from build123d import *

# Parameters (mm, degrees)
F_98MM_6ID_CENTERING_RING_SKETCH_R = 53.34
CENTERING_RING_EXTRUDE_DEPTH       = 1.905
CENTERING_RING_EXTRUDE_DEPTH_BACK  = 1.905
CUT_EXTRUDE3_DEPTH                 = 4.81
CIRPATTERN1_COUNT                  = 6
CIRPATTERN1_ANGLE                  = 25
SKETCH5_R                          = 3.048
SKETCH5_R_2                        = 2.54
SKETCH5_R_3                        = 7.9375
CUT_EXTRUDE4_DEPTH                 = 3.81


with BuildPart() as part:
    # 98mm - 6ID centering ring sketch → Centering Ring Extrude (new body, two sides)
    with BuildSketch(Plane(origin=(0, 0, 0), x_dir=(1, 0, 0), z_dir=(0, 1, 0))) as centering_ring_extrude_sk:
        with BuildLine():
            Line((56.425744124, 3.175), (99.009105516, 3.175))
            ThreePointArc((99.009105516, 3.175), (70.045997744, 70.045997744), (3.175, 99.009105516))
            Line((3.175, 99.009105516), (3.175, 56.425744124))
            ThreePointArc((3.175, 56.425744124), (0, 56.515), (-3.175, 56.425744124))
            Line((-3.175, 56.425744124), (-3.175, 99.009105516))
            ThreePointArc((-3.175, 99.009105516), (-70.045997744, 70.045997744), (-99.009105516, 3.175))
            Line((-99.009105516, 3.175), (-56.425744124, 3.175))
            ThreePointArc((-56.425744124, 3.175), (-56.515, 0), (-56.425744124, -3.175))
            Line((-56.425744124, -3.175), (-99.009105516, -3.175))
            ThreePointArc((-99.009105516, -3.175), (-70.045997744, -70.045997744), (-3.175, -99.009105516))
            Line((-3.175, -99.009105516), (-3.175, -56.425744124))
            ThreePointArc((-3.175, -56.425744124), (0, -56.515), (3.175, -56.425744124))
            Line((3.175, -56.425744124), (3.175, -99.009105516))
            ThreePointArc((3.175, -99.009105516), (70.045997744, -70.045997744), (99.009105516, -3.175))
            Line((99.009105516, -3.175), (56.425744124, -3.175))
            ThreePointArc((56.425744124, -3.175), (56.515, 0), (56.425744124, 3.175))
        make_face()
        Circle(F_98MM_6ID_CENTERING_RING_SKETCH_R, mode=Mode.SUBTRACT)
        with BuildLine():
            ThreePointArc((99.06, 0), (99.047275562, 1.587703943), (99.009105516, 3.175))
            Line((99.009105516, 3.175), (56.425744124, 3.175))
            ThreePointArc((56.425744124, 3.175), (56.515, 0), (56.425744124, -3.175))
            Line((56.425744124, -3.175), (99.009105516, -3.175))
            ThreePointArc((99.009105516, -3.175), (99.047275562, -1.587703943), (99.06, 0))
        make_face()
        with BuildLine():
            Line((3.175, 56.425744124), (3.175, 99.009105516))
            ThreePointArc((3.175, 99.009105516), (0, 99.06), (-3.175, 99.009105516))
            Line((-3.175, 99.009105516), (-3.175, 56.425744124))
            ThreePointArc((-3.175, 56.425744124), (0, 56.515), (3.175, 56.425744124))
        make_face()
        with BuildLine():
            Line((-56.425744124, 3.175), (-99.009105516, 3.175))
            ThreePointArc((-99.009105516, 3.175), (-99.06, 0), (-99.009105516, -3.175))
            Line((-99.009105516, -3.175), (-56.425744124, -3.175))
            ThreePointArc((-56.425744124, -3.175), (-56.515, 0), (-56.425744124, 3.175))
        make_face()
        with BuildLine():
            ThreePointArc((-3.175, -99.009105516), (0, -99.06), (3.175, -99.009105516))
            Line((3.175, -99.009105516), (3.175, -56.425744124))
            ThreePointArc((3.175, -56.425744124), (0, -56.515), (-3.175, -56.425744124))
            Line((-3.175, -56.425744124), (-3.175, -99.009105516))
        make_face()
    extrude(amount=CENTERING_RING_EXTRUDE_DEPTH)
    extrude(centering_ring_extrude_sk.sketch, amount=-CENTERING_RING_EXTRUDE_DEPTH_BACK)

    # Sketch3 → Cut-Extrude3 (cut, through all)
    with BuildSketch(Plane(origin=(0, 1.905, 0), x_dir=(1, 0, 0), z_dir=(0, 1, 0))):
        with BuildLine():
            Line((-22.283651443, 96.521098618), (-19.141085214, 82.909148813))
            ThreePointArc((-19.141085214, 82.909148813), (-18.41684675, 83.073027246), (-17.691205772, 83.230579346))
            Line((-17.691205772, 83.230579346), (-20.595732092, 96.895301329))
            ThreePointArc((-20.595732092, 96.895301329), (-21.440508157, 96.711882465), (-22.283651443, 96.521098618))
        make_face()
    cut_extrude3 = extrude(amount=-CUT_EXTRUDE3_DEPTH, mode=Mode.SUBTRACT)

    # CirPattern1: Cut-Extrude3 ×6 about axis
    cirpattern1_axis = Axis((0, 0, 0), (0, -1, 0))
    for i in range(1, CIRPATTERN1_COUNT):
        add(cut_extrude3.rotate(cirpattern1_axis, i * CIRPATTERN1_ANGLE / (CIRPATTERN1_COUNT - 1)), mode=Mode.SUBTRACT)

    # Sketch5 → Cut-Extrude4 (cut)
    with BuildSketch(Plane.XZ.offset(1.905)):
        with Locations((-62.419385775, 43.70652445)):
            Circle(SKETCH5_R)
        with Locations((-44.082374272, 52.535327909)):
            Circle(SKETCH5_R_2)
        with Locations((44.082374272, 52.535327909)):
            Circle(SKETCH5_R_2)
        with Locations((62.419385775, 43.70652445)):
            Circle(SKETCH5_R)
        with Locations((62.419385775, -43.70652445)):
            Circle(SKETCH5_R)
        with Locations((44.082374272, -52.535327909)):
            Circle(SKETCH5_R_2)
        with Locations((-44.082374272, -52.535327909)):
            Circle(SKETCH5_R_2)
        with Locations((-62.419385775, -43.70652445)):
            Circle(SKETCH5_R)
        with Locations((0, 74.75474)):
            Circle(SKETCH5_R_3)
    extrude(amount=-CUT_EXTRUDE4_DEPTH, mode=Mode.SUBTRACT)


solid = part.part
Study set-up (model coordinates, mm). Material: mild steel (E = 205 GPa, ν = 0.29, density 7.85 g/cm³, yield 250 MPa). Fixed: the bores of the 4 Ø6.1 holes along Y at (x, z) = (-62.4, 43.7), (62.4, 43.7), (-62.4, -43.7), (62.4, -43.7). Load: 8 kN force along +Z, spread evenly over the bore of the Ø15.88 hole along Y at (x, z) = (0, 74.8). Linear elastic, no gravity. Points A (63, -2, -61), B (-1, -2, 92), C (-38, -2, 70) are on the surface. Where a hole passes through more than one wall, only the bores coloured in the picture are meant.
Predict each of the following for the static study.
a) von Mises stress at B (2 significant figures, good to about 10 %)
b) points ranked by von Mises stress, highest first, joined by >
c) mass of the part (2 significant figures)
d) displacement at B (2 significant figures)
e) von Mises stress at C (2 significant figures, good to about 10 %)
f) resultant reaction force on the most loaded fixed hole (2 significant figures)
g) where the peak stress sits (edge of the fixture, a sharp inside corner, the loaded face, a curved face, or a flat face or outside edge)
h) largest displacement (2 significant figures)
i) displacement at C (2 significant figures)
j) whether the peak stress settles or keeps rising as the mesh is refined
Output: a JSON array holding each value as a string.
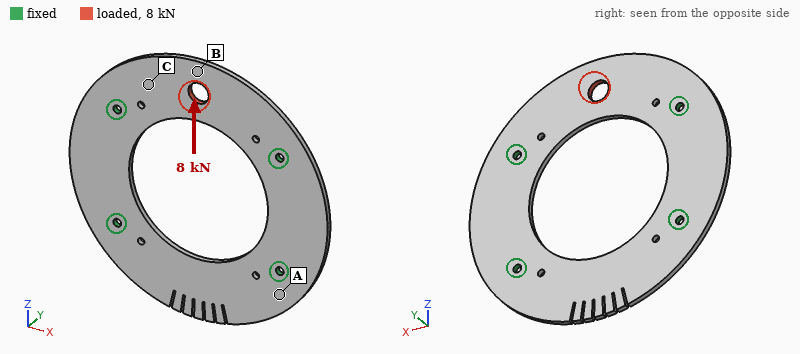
["68 MPa", "B > C > A", "640 g", "27 µm", "37 MPa", "4.9 kN", "edge of the fixture", "31 µm", "12 µm", "keeps rising"]
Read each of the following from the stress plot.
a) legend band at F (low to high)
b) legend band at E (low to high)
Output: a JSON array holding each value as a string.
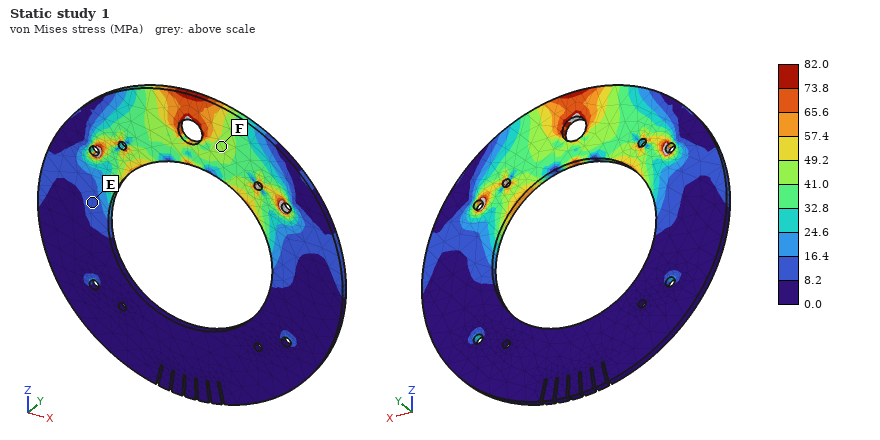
["41.0 to 49.2 MPa", "8.2 to 16.4 MPa"]
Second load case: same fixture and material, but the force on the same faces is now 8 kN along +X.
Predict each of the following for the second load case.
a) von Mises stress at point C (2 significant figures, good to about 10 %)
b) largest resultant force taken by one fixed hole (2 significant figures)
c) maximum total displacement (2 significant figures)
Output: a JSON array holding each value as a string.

["25 MPa", "4.4 kN", "18 µm"]
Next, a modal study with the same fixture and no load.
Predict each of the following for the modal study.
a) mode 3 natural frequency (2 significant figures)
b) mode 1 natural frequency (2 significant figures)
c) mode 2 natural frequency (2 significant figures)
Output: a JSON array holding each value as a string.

["1700 Hz", "740 Hz", "760 Hz"]
